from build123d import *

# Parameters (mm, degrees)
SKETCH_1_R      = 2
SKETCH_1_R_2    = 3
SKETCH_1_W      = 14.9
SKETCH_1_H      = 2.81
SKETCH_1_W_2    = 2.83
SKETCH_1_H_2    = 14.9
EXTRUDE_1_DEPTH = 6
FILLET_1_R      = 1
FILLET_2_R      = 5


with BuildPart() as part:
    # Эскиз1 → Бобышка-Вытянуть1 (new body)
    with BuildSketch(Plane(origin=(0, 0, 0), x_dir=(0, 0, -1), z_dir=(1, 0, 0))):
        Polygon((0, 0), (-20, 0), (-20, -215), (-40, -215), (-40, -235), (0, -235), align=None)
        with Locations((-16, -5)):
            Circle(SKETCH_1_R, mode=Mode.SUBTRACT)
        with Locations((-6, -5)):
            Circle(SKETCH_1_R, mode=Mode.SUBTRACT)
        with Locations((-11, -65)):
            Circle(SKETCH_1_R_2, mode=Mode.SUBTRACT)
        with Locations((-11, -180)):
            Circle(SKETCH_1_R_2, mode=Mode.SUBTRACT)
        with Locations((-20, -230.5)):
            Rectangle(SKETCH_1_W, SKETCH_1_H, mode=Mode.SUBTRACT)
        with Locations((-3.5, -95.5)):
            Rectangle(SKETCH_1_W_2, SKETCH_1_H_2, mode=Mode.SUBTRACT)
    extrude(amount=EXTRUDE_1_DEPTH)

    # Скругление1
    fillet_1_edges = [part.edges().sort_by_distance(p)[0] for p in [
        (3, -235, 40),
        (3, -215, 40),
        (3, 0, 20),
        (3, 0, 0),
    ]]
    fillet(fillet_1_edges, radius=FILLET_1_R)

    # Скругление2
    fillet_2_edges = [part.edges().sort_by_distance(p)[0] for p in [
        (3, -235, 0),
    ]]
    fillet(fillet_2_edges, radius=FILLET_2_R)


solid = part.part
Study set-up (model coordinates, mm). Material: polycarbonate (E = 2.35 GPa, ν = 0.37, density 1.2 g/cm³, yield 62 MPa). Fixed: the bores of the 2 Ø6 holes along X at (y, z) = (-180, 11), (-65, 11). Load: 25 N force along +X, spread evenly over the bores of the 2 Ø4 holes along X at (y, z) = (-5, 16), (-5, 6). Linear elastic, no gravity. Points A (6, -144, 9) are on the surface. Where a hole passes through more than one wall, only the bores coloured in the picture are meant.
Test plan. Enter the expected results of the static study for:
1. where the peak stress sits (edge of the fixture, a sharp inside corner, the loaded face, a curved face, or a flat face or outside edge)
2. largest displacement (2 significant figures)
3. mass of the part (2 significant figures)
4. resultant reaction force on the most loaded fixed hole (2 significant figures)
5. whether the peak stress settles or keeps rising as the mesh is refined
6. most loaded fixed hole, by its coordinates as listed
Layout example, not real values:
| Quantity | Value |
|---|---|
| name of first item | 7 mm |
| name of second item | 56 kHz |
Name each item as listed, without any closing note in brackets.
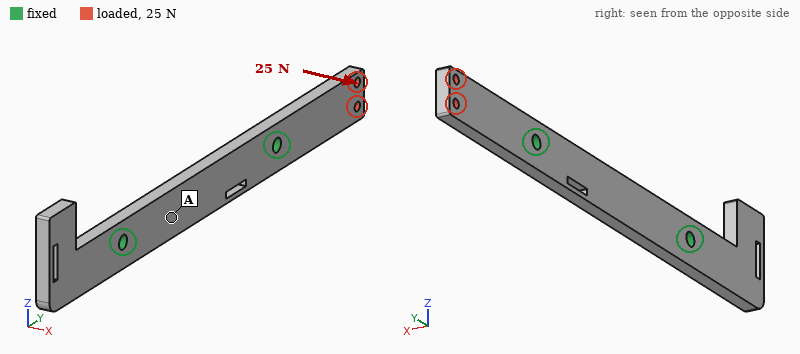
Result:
| Quantity | Value |
|---|---|
| where the peak stress sits | edge of the fixture |
| largest displacement | 2.3 mm |
| mass of the part | 35 g |
| resultant reaction force on the most loaded fixed hole | 25 N |
| whether the peak stress settles or keeps rising as the mesh is refined | keeps rising |
| most loaded fixed hole, by its coordinates as listed | (-65, 11) |
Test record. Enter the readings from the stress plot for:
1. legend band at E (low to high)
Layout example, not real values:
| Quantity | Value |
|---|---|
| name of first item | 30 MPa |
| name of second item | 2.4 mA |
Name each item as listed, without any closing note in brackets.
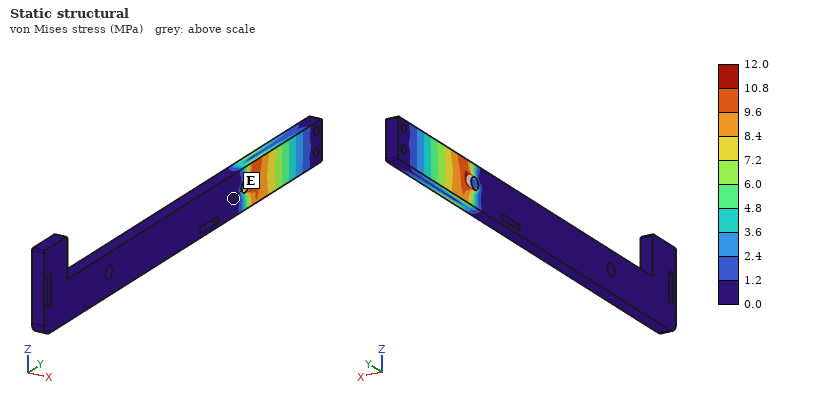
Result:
| Quantity | Value |
|---|---|
| legend band at E | 0.0 to 1.2 MPa |
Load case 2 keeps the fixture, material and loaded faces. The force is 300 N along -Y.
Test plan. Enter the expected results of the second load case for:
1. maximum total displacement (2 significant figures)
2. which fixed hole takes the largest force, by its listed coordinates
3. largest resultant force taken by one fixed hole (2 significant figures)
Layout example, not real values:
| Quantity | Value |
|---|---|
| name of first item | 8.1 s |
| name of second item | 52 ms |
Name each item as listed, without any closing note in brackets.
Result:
| Quantity | Value |
|---|---|
| maximum total displacement | 0.10 mm |
| which fixed hole takes the largest force, by its listed coordinates | (-65, 11) |
| largest resultant force taken by one fixed hole | 290 N |
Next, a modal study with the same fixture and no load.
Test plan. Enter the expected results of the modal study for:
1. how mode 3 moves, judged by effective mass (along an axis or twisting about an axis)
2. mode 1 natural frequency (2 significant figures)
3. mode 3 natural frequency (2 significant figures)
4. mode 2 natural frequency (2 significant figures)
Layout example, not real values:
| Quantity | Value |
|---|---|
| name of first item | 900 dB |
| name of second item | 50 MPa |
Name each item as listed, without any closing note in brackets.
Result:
| Quantity | Value |
|---|---|
| how mode 3 moves, judged by effective mass | along X |
| mode 1 natural frequency | 340 Hz |
| mode 3 natural frequency | 670 Hz |
| mode 2 natural frequency | 340 Hz |
